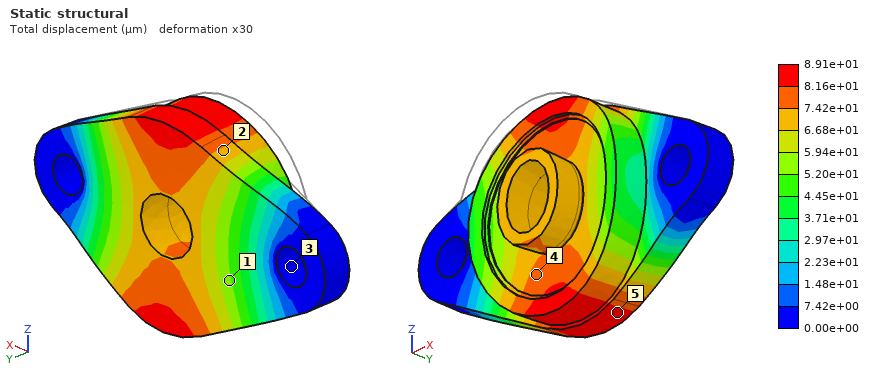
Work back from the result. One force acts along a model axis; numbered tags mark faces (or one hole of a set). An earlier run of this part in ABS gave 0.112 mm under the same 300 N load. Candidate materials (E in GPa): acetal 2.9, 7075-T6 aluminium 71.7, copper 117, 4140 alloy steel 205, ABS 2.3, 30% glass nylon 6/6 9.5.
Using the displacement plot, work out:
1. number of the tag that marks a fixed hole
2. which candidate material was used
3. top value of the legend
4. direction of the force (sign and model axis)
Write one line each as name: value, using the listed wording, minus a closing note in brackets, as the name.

number of the tag that marks a fixed hole: 3
which candidate material was used: acetal
top value of the legend: 8.91e+01 µm
direction of the force: +Y
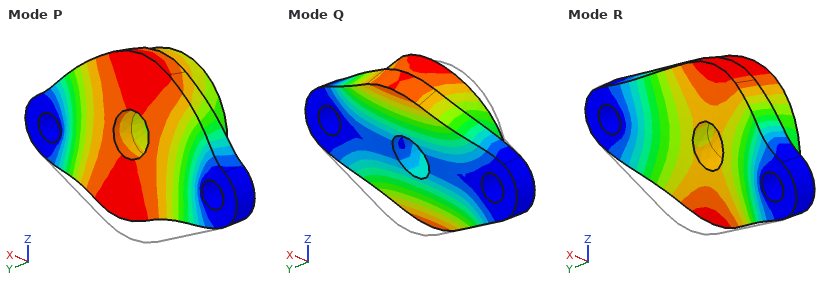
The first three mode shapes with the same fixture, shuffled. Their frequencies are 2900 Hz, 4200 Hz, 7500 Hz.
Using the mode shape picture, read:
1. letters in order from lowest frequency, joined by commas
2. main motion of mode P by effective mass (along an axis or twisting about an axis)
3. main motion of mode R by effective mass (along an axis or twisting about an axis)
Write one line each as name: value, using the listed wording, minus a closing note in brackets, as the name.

letters in order from lowest frequency, joined by commas: Q, R, P
main motion of mode P by effective mass: along Z
main motion of mode R by effective mass: along Y
